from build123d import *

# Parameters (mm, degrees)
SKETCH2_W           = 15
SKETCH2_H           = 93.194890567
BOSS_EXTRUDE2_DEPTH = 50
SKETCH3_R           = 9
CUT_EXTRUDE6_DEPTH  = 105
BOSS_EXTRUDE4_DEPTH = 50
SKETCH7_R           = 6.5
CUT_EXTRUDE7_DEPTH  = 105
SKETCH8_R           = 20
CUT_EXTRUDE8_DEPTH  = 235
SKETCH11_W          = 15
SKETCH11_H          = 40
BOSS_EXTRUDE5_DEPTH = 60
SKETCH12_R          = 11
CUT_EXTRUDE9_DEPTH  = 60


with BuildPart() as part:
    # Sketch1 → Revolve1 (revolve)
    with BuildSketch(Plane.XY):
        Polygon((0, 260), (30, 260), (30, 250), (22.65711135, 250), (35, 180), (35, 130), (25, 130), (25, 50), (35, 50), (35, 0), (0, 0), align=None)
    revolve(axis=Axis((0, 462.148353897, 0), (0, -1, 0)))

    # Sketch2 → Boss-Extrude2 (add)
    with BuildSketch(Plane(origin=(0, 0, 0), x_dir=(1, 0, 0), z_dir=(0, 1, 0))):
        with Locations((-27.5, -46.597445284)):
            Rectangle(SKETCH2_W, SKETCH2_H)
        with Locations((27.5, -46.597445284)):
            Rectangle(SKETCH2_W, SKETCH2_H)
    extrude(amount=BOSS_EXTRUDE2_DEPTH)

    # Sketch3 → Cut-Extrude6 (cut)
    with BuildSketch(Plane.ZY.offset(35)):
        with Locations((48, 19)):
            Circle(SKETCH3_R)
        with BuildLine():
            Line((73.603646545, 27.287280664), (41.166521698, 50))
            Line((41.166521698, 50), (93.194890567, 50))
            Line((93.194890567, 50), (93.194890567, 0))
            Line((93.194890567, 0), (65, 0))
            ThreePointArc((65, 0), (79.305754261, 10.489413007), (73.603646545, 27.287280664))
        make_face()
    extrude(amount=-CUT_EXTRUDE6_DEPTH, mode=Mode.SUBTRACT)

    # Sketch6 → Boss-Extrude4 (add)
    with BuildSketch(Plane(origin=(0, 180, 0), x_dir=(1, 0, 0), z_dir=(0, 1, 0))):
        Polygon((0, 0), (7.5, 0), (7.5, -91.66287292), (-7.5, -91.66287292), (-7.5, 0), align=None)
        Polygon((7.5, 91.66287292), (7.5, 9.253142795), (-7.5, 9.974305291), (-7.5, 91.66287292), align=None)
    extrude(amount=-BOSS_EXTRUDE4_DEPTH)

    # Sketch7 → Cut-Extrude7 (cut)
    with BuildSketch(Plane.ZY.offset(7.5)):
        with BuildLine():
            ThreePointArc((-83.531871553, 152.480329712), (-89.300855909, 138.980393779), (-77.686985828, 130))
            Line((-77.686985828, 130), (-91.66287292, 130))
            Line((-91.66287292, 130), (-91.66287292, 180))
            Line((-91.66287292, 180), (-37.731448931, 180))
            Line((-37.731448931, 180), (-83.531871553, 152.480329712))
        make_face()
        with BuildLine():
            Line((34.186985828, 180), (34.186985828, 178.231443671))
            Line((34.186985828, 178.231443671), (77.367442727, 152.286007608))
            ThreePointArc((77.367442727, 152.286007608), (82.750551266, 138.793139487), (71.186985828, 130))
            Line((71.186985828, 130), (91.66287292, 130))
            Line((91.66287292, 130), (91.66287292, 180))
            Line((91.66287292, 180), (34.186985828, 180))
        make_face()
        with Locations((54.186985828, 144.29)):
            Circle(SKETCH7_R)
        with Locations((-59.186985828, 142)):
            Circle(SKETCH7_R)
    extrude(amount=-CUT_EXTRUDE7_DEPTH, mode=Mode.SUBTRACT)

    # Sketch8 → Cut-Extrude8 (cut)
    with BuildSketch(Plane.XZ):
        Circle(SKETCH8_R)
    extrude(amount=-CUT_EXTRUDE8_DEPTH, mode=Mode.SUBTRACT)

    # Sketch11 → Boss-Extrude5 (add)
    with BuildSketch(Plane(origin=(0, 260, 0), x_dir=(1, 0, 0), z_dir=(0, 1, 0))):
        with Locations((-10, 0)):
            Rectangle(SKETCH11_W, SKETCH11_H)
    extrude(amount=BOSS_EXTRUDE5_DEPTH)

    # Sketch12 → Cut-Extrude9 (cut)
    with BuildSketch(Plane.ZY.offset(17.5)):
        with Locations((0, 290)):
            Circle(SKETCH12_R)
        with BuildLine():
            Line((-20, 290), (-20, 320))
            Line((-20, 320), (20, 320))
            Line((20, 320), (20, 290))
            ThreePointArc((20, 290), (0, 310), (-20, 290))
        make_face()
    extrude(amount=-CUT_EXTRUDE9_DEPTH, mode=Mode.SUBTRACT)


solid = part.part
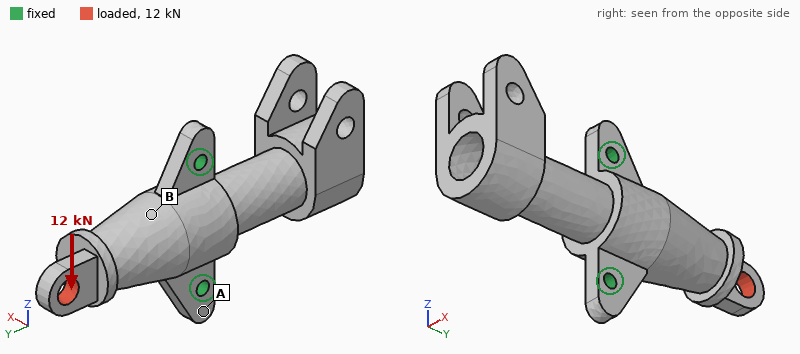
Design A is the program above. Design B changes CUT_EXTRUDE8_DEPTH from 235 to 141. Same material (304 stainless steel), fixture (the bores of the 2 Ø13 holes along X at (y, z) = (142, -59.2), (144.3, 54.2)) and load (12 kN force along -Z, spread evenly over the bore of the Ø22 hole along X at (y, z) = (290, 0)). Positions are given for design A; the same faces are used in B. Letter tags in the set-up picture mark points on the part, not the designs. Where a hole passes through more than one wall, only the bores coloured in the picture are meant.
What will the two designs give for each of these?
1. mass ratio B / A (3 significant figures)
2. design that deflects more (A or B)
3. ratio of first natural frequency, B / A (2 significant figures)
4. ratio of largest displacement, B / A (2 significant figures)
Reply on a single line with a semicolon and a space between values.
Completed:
1.20; A; 0.98; 0.87
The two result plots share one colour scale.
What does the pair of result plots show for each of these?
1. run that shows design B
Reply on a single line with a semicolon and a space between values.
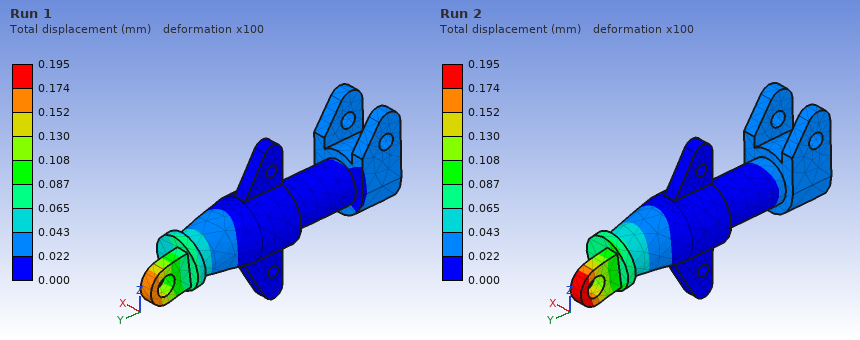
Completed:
Run 1
